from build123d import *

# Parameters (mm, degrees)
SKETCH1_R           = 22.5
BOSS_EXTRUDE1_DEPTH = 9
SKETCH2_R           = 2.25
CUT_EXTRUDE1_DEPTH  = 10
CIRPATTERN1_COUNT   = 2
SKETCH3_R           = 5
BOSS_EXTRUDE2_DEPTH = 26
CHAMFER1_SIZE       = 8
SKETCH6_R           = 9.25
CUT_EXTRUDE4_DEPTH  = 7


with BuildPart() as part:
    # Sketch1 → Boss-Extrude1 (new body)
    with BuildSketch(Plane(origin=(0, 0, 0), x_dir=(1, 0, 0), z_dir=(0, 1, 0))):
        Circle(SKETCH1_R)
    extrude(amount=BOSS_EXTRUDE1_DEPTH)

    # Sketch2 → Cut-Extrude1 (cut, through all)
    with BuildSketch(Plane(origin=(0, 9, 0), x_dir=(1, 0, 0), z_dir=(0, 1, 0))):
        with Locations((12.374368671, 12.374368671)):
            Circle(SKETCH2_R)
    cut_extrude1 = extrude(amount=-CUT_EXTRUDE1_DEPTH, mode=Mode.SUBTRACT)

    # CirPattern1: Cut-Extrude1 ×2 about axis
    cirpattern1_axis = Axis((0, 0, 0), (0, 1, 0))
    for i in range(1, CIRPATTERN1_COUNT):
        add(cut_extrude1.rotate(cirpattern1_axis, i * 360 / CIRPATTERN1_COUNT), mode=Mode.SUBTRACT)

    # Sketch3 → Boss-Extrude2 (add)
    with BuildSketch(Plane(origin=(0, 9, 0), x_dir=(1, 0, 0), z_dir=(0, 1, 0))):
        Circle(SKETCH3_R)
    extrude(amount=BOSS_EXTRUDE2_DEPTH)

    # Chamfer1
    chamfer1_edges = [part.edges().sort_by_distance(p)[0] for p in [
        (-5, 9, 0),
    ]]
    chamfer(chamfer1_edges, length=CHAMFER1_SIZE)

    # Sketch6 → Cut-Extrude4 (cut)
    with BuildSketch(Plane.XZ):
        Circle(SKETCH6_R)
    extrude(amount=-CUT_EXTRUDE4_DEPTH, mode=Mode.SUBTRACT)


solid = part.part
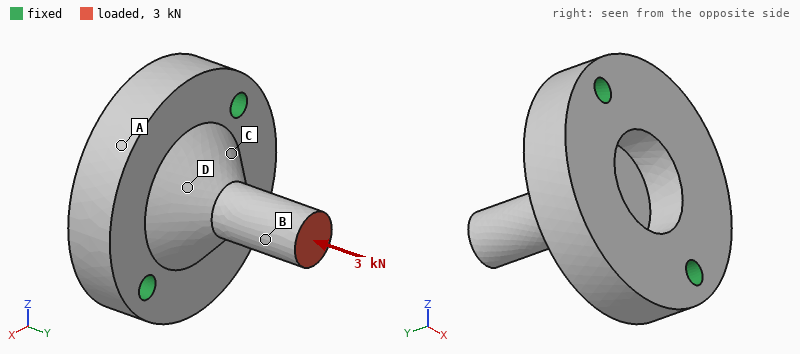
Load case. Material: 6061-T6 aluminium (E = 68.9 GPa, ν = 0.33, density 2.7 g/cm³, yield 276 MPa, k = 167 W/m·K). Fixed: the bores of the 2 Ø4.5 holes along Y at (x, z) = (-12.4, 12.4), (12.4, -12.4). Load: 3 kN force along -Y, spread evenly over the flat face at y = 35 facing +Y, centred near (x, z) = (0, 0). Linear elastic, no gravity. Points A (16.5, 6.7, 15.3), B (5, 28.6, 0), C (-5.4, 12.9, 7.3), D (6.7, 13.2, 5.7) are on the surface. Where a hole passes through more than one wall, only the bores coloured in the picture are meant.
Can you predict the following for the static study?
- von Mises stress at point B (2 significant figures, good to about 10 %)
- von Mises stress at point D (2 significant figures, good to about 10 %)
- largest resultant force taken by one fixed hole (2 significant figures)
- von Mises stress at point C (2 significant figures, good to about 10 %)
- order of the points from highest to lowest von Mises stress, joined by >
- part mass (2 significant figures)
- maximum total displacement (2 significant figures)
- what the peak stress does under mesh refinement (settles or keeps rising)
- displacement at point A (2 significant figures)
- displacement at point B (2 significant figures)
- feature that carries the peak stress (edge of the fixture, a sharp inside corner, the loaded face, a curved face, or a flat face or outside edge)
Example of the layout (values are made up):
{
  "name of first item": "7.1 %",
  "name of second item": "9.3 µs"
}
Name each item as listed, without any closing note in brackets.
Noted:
{
  "von Mises stress at point B": "38 MPa",
  "von Mises stress at point D": "11 MPa",
  "largest resultant force taken by one fixed hole": "1.7 kN",
  "von Mises stress at point C": "29 MPa",
  "order of the points from highest to lowest von Mises stress, joined by >": "B > C > D > A",
  "part mass": "42 g",
  "maximum total displacement": "20 µm",
  "what the peak stress does under mesh refinement": "keeps rising",
  "displacement at point A": "9.0 µm",
  "displacement at point B": "16 µm",
  "feature that carries the peak stress": "edge of the fixture"
}
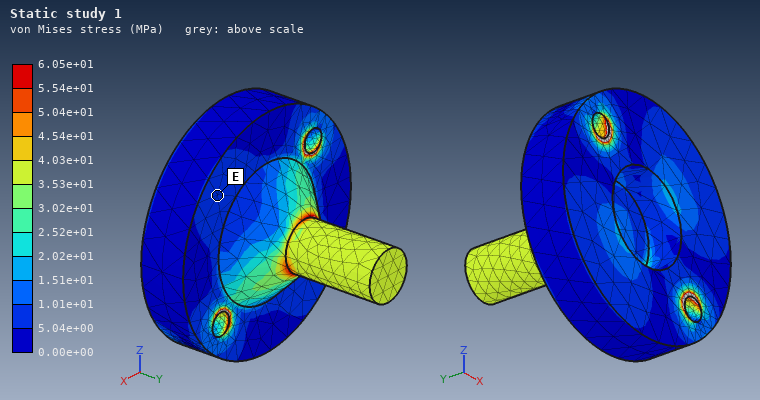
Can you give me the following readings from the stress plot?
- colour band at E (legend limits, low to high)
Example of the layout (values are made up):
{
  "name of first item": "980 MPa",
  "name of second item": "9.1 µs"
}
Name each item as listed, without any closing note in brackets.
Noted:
{
  "colour band at E": "5.04e+00 to 1.01e+01 MPa"
}
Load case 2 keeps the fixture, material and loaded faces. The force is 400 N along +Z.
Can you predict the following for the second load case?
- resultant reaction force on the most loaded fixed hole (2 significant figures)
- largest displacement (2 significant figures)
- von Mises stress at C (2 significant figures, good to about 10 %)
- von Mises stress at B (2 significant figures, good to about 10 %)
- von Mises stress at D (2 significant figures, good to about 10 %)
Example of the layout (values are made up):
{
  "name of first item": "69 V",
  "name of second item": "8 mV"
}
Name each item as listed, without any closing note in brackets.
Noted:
{
  "resultant reaction force on the most loaded fixed hole": "350 N",
  "largest displacement": "52 µm",
  "von Mises stress at C": "15 MPa",
  "von Mises stress at B": "11 MPa",
  "von Mises stress at D": "10 MPa"
}
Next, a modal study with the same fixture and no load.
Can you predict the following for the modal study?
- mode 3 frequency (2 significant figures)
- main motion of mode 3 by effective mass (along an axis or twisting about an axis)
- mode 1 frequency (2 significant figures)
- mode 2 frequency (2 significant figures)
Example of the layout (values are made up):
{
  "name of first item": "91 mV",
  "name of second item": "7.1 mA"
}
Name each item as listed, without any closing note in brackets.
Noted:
{
  "mode 3 frequency": "16 kHz",
  "main motion of mode 3 by effective mass": "along Y",
  "mode 1 frequency": "9000 Hz",
  "mode 2 frequency": "14 kHz"
}
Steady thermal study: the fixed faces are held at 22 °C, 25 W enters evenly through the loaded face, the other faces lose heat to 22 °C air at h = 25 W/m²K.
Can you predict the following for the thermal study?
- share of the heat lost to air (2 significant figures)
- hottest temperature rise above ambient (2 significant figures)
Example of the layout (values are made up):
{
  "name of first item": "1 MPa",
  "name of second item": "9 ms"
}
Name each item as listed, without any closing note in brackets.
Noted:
{
  "share of the heat lost to air": "3.3 %",
  "hottest temperature rise above ambient": "47 K"
}
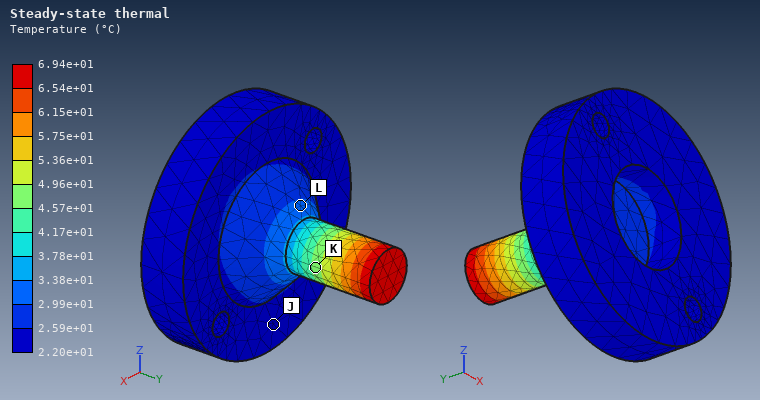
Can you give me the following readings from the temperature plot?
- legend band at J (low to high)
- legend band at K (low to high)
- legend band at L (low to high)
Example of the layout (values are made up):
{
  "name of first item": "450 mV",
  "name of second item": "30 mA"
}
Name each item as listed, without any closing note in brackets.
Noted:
{
  "legend band at J": "2.20e+01 to 2.59e+01 °C",
  "legend band at K": "4.57e+01 to 4.96e+01 °C",
  "legend band at L": "2.99e+01 to 3.38e+01 °C"
}
